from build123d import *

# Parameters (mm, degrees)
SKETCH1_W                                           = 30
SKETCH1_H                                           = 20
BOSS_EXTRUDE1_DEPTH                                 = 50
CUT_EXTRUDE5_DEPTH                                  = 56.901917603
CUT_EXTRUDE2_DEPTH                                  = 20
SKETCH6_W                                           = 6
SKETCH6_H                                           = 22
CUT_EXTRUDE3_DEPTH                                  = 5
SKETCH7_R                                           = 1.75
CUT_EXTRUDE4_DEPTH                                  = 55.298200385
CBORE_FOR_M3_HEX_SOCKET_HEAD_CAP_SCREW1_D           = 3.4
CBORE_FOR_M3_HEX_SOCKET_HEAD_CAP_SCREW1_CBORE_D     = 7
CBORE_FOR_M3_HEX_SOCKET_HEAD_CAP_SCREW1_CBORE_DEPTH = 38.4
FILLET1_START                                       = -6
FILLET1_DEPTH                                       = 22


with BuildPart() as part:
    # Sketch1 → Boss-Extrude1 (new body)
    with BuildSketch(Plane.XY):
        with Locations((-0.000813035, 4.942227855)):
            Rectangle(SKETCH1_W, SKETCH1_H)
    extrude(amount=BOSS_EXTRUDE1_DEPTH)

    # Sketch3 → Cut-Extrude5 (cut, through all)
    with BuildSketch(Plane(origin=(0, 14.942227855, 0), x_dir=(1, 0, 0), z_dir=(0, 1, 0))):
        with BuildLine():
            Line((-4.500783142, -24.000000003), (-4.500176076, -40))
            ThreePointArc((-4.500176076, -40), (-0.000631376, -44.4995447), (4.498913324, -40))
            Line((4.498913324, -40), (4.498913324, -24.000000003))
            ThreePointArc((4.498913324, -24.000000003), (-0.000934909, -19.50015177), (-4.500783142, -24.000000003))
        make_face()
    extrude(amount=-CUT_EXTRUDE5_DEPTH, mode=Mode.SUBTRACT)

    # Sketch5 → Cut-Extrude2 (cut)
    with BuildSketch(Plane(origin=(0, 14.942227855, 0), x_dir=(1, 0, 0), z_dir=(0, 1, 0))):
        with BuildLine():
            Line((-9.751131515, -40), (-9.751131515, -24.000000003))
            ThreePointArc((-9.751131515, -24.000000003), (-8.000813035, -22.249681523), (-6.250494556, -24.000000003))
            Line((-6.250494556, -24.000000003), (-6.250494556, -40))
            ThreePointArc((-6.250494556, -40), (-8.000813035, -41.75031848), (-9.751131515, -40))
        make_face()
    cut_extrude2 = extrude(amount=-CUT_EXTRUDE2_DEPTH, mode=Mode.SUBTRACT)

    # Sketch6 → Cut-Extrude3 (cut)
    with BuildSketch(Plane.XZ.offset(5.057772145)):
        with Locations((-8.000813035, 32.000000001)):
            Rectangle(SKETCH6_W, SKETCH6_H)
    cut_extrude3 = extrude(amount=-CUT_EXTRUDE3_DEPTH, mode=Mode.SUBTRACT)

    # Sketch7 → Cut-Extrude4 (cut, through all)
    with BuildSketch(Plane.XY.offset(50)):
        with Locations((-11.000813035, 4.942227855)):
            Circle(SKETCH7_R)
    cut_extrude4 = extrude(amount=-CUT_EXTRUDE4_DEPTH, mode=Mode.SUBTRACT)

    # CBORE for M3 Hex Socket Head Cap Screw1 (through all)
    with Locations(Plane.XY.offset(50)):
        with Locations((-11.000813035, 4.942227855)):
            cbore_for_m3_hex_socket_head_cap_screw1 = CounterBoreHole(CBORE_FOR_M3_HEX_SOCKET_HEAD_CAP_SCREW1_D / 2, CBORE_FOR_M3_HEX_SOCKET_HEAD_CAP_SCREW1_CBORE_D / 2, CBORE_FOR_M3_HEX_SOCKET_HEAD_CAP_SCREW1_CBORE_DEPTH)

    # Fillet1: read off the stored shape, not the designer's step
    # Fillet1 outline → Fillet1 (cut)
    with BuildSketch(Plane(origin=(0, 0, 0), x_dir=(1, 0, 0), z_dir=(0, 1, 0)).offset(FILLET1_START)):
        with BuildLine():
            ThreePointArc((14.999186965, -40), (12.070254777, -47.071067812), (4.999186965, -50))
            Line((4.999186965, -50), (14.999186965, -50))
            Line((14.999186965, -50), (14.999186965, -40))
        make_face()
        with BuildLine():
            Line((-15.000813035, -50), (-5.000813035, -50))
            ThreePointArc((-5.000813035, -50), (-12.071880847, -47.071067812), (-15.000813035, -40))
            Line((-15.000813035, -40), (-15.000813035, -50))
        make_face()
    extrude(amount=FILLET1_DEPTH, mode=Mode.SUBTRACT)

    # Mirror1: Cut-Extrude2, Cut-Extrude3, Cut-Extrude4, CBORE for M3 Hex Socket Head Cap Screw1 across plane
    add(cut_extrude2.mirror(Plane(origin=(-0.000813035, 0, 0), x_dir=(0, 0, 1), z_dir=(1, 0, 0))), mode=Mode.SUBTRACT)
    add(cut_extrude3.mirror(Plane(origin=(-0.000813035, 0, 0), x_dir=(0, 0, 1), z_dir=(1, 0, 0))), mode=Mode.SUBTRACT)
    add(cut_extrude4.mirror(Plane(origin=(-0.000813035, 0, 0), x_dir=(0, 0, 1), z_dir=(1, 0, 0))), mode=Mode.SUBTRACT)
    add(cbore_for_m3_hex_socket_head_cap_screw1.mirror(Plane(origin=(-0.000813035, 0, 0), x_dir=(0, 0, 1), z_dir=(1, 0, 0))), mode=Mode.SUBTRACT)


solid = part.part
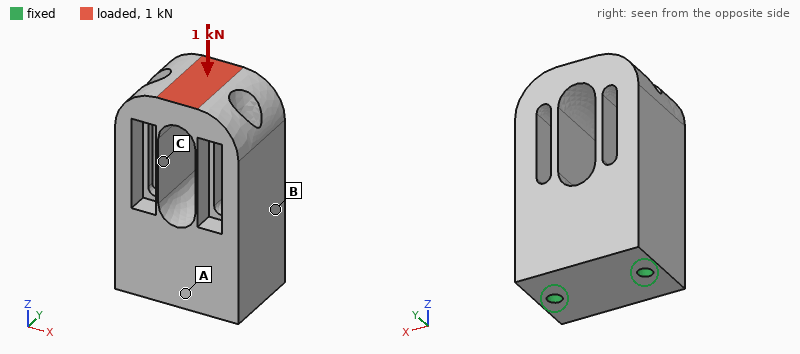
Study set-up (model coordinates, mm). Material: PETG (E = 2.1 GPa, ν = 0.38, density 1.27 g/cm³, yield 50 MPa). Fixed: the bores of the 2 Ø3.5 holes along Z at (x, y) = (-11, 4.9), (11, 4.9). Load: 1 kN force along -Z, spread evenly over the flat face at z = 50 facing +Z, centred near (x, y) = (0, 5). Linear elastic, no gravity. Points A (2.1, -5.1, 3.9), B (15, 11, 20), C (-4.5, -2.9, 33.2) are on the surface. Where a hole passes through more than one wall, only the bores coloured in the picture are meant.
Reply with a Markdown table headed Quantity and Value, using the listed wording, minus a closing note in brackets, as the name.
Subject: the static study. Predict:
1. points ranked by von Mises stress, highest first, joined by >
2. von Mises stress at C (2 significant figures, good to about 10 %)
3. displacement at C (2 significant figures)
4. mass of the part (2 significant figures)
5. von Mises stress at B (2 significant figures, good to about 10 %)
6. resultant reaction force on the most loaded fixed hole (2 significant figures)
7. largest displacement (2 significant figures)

| Quantity | Value |
|---|---|
| points ranked by von Mises stress, highest first, joined by > | C > B > A |
| von Mises stress at C | 16 MPa |
| displacement at C | 0.15 mm |
| mass of the part | 24 g |
| von Mises stress at B | 4.4 MPa |
| resultant reaction force on the most loaded fixed hole | 500 N |
| largest displacement | 0.27 mm |
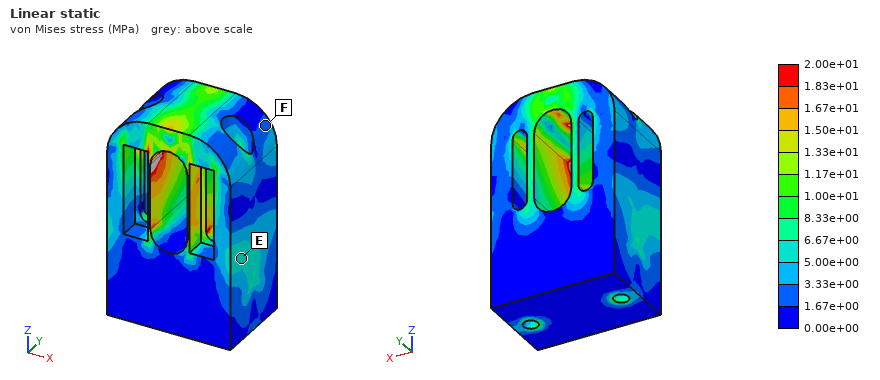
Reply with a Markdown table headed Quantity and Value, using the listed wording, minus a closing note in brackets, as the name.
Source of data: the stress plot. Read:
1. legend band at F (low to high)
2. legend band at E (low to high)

| Quantity | Value |
|---|---|
| legend band at F | 1.67e+00 to 3.33e+00 MPa |
| legend band at E | 5.00e+00 to 6.67e+00 MPa |
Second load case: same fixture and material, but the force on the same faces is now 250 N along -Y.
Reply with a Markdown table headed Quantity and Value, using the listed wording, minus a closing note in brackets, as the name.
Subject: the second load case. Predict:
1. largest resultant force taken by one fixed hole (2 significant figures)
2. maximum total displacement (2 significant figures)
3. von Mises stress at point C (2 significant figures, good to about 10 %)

| Quantity | Value |
|---|---|
| largest resultant force taken by one fixed hole | 130 N |
| maximum total displacement | 0.73 mm |
| von Mises stress at point C | 9.4 MPa |
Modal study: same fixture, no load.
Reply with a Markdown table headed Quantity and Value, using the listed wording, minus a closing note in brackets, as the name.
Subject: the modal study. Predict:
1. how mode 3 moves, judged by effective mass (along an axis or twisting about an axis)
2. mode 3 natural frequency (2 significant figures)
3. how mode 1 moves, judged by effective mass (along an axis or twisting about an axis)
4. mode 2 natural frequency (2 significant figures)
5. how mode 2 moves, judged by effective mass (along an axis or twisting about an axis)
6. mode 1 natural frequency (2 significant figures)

| Quantity | Value |
|---|---|
| how mode 3 moves, judged by effective mass | twisting about Z |
| mode 3 natural frequency | 2600 Hz |
| how mode 1 moves, judged by effective mass | along X |
| mode 2 natural frequency | 1400 Hz |
| how mode 2 moves, judged by effective mass | along Y |
| mode 1 natural frequency | 1300 Hz |
